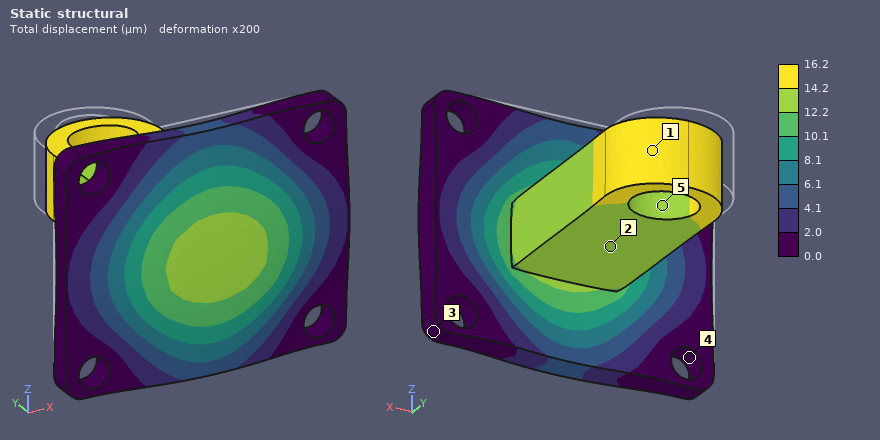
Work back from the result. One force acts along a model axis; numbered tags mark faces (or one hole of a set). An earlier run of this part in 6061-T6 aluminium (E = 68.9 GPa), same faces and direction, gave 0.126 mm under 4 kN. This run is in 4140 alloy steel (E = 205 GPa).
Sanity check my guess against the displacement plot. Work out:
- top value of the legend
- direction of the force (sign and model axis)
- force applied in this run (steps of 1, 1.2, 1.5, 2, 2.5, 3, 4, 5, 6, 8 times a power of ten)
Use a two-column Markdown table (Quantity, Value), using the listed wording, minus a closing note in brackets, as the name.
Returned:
| Quantity | Value |
|---|---|
| top value of the legend | 16.2 µm |
| direction of the force | -Y |
| force applied in this run | 1.5 kN |
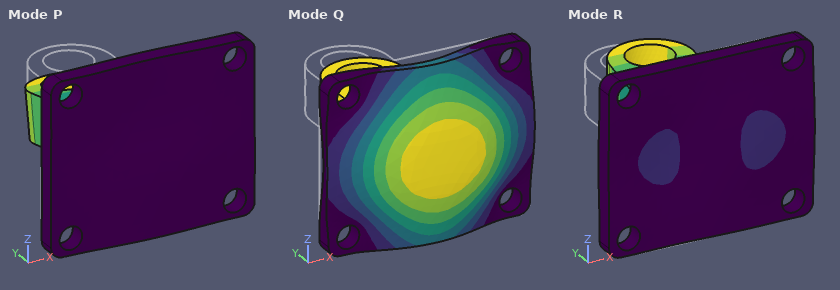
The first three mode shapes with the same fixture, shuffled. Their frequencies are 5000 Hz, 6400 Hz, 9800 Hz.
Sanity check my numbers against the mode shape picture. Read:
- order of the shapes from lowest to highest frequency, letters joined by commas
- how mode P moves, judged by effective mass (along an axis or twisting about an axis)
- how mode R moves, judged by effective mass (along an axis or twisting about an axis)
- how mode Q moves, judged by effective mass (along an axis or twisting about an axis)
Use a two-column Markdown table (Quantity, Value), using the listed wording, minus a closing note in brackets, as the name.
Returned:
| Quantity | Value |
|---|---|
| order of the shapes from lowest to highest frequency, letters joined by commas | P, R, Q |
| how mode P moves, judged by effective mass | along Z |
| how mode R moves, judged by effective mass | along X |
| how mode Q moves, judged by effective mass | along Y |
